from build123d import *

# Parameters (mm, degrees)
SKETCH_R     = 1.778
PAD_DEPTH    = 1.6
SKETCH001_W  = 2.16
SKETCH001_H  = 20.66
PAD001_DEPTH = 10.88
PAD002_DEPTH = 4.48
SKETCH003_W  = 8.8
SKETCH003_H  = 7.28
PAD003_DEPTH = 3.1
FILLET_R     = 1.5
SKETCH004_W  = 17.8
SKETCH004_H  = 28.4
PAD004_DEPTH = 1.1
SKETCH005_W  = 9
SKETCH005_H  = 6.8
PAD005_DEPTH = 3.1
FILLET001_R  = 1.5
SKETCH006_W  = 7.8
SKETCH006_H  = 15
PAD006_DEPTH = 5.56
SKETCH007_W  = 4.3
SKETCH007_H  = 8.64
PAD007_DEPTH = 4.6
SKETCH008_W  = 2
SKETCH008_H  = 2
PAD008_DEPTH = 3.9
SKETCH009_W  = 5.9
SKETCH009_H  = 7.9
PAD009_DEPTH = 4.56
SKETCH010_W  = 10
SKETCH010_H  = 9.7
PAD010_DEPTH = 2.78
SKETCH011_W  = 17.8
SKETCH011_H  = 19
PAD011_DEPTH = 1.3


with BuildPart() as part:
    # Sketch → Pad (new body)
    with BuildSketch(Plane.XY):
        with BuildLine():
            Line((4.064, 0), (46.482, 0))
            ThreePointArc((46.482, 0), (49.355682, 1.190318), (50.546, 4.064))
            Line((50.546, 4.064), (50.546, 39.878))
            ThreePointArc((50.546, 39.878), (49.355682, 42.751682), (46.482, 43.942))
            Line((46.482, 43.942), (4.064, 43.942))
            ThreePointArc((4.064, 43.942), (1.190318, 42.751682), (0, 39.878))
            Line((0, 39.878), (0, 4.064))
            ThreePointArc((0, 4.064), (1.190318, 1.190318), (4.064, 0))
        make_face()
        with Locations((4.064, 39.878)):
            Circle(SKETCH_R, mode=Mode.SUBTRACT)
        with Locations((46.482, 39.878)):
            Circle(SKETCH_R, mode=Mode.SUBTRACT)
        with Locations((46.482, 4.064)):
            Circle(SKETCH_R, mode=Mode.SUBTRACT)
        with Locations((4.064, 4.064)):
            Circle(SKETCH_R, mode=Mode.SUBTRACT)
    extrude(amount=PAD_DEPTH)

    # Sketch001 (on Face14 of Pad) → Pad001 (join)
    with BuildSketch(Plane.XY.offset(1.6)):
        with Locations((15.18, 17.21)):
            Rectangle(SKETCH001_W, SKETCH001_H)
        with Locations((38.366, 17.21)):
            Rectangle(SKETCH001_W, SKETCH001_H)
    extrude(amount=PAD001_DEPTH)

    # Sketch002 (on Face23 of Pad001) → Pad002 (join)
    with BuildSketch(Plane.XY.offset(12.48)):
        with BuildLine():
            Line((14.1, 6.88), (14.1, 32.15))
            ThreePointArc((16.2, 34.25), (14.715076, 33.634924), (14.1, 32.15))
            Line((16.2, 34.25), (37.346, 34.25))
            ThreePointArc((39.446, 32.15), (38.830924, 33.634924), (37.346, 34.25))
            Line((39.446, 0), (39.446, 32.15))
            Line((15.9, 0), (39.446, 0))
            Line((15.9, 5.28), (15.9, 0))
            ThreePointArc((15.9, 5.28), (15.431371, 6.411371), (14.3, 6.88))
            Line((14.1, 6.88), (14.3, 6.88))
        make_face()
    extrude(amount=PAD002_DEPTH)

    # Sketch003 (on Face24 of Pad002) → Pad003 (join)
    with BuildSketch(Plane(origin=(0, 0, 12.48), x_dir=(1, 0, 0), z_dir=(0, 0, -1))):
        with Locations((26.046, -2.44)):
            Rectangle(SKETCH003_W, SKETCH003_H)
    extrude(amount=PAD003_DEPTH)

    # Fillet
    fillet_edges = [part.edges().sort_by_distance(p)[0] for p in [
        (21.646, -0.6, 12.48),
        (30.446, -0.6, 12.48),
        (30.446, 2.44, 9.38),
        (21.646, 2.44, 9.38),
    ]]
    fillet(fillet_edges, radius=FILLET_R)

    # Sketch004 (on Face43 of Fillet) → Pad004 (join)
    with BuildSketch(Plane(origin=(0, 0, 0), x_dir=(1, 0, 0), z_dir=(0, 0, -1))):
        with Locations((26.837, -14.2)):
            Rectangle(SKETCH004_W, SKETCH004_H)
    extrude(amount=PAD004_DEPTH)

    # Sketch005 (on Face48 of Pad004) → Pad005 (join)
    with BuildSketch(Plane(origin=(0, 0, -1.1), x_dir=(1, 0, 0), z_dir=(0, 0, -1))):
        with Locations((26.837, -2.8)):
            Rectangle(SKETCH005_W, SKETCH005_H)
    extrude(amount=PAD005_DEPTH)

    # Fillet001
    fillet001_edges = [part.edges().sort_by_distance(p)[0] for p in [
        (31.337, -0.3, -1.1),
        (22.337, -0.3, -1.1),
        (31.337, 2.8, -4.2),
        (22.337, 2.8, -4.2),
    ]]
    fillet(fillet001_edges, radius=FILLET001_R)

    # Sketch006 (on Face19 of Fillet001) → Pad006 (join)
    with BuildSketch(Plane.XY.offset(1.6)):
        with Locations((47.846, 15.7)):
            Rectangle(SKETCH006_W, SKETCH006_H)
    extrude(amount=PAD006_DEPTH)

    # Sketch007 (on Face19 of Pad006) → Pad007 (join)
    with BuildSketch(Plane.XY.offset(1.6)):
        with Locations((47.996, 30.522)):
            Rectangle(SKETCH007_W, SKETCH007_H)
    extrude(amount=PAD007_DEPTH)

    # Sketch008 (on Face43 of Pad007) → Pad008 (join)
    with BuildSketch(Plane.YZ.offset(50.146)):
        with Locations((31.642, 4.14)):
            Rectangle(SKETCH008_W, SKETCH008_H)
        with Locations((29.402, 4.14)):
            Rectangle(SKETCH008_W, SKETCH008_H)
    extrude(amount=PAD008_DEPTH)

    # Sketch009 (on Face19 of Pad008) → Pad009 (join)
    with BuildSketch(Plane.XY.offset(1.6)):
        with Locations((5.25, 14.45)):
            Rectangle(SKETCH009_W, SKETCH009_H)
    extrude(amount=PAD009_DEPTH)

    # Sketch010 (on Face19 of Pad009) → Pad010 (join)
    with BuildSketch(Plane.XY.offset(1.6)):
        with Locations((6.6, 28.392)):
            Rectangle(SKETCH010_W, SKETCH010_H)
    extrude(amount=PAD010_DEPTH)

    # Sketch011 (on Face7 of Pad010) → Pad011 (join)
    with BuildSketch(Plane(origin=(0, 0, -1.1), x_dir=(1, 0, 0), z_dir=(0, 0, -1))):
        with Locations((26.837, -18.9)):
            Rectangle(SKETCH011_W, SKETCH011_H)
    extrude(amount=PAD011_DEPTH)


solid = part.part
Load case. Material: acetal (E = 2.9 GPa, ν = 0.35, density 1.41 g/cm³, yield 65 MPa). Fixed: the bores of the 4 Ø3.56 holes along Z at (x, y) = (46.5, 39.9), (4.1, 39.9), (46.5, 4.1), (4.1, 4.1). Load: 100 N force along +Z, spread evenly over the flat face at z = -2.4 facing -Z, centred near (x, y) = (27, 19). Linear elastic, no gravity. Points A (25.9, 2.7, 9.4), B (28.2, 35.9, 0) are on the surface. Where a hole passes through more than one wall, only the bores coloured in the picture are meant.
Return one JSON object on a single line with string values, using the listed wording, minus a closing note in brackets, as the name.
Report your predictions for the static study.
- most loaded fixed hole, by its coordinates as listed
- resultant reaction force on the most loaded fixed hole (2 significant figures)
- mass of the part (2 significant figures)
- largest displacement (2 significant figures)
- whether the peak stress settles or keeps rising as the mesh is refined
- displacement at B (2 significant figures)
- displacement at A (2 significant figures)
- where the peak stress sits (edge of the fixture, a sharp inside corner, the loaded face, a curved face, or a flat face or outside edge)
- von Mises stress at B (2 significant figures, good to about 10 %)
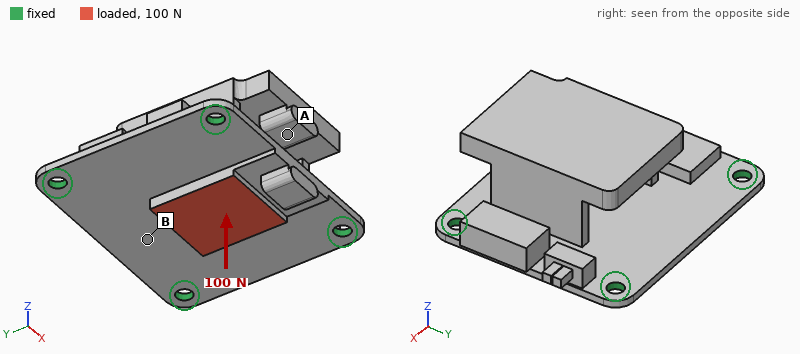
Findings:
{"most loaded fixed hole, by its coordinates as listed": "(46.5, 4.1)", "resultant reaction force on the most loaded fixed hole": "35 N", "mass of the part": "15 g", "largest displacement": "0.45 mm", "whether the peak stress settles or keeps rising as the mesh is refined": "keeps rising", "displacement at B": "0.35 mm", "displacement at A": "0.18 mm", "where the peak stress sits": "edge of the fixture", "von Mises stress at B": "5.1 MPa"}
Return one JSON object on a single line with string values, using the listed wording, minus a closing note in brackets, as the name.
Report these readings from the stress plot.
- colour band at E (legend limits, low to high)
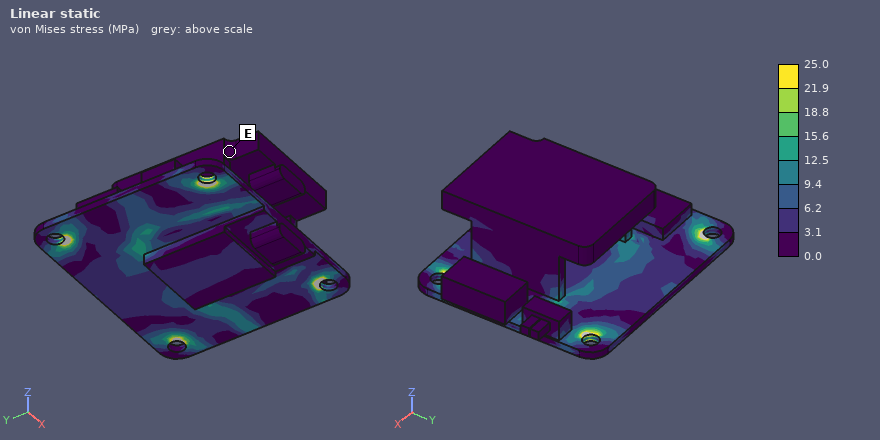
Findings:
{"colour band at E": "0.0 to 3.1 MPa"}
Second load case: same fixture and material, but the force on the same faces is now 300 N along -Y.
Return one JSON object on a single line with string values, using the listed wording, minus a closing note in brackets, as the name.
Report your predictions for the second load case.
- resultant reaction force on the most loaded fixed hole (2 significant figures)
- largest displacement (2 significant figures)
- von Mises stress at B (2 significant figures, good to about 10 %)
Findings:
{"resultant reaction force on the most loaded fixed hole": "100 N", "largest displacement": "0.33 mm", "von Mises stress at B": "5.6 MPa"}
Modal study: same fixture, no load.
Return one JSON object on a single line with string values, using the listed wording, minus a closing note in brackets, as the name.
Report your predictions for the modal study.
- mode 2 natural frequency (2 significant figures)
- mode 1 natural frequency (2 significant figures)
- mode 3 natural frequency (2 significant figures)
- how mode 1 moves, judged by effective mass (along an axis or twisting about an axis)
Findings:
{"mode 2 natural frequency": "950 Hz", "mode 1 natural frequency": "800 Hz", "mode 3 natural frequency": "1100 Hz", "how mode 1 moves, judged by effective mass": "along Z"}
